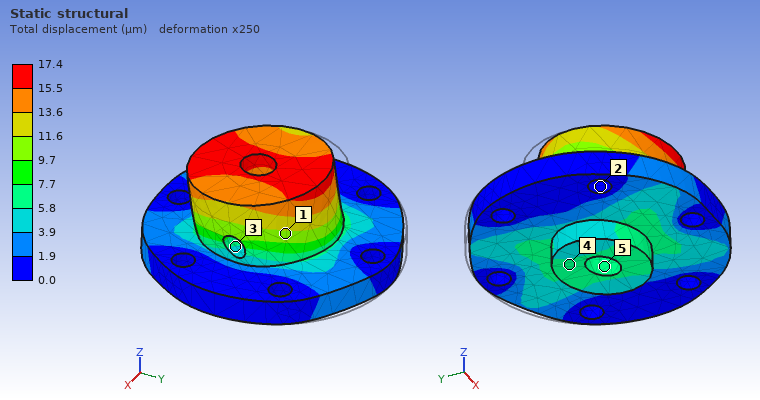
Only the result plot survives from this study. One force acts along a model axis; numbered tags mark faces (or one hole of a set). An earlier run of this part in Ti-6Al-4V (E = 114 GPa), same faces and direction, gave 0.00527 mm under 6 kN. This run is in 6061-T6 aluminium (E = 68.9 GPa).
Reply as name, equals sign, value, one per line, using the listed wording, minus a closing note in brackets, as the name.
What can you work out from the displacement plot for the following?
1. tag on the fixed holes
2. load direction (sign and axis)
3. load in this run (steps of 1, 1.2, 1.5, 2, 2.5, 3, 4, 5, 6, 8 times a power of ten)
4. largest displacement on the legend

tag on the fixed holes = 2
load direction = -Y
load in this run = 12 kN
largest displacement on the legend = 17.4 µm
